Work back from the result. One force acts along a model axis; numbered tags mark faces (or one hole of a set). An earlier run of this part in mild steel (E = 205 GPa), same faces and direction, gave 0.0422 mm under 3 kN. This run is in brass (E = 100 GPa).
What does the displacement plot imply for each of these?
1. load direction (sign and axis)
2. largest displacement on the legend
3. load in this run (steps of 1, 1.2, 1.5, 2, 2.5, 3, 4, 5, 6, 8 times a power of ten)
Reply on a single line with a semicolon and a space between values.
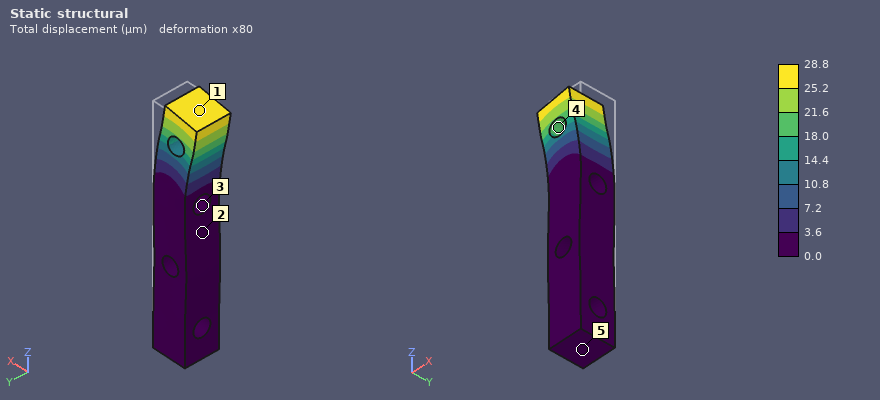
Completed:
-X; 28.8 µm; 1 kN
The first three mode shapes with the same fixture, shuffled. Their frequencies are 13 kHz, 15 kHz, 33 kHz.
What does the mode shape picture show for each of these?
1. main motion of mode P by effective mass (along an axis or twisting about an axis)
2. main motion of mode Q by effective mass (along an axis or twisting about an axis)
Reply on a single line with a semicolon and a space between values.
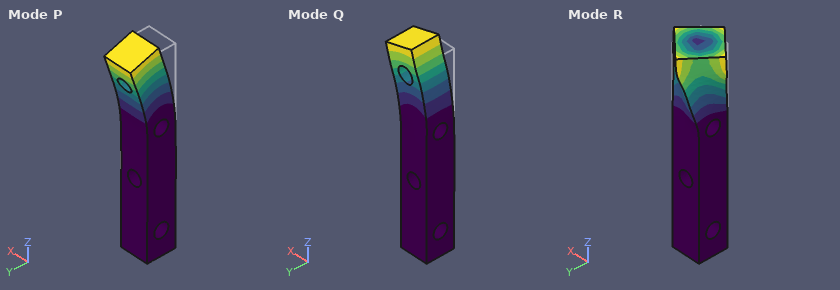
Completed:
along Y; along X
